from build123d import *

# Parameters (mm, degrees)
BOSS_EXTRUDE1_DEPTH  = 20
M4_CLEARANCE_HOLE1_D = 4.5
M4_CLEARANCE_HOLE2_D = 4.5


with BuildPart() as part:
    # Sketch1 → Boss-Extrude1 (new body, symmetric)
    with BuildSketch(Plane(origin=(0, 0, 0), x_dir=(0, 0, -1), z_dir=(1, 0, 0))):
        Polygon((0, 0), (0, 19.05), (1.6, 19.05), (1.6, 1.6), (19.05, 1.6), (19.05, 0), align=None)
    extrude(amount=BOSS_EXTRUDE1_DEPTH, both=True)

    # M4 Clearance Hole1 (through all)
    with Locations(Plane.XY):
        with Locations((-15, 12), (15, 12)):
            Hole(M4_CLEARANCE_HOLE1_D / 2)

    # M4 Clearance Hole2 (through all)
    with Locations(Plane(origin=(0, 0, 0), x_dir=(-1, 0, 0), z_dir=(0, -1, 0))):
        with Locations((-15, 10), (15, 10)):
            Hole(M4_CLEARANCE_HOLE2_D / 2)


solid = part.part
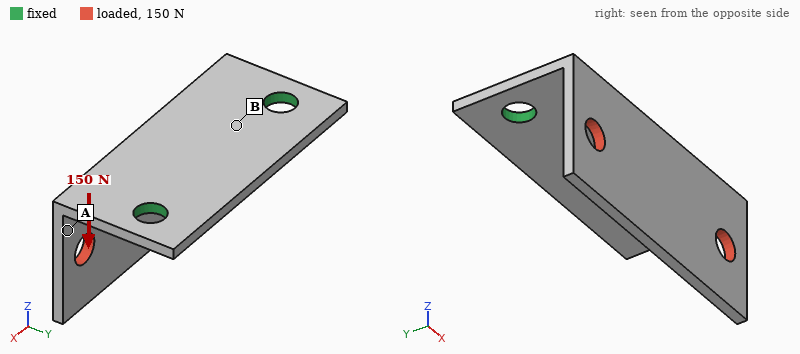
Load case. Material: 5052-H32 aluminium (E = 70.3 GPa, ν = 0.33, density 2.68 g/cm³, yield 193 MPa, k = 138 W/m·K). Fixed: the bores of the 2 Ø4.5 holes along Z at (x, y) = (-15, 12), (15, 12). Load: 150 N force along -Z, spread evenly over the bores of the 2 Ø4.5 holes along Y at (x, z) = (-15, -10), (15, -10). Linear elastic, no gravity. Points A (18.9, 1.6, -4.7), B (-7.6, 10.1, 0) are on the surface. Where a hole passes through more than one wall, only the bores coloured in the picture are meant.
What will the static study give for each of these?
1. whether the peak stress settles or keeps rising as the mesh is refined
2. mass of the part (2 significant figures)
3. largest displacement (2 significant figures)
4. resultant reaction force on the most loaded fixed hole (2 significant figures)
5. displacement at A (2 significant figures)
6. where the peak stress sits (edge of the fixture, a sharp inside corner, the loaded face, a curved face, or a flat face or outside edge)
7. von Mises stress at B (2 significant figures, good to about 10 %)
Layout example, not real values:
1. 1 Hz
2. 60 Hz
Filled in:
1. keeps rising
2. 6.0 g
3. 0.17 mm
4. 75 N
5. 0.068 mm
6. edge of the fixture
7. 37 MPa
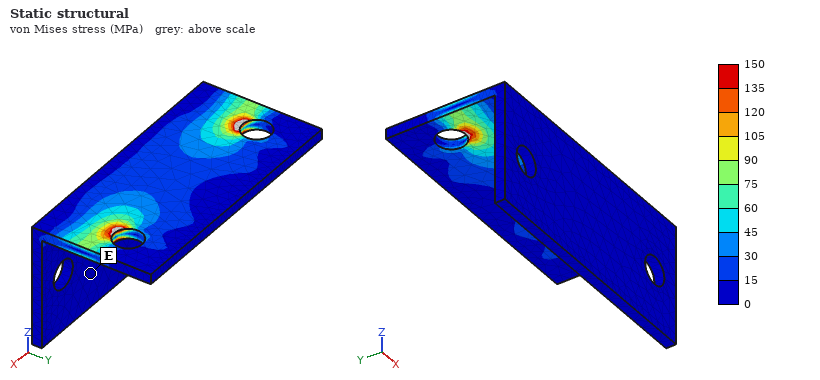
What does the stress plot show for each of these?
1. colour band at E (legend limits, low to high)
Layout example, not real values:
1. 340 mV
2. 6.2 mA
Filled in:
1. 0 to 15 MPa
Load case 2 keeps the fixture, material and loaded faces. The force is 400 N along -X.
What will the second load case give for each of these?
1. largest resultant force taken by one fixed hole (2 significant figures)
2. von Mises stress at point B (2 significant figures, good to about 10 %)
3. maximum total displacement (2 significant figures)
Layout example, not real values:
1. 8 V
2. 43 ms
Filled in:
1. 270 N
2. 22 MPa
3. 0.16 mm
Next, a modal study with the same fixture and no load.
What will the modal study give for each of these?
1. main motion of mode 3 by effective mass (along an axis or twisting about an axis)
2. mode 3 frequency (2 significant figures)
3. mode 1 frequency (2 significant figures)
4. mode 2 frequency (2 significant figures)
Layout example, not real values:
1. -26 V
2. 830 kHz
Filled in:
1. along Z
2. 6100 Hz
3. 2100 Hz
4. 4000 Hz
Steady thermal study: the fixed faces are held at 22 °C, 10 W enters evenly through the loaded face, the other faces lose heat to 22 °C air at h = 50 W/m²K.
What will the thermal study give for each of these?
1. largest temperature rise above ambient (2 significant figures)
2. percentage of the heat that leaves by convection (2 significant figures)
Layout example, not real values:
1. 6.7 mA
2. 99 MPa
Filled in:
1. 27 K
2. 18 %
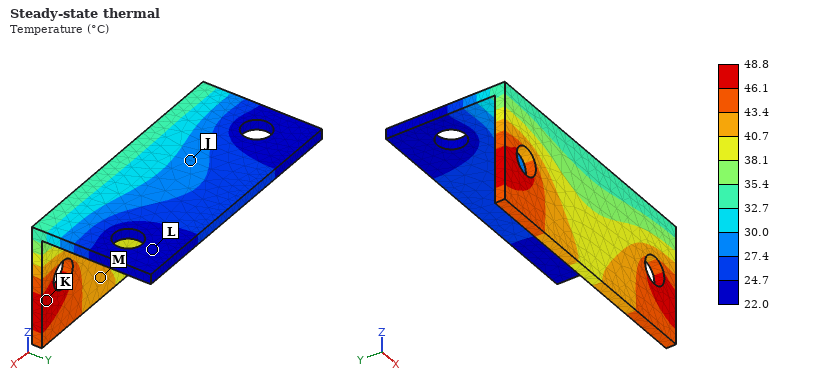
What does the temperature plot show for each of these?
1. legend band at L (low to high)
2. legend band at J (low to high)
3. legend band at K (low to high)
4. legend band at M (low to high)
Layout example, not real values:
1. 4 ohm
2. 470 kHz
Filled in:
1. 22.0 to 24.7 °C
2. 27.4 to 30.0 °C
3. 46.1 to 48.8 °C
4. 40.7 to 43.4 °C
